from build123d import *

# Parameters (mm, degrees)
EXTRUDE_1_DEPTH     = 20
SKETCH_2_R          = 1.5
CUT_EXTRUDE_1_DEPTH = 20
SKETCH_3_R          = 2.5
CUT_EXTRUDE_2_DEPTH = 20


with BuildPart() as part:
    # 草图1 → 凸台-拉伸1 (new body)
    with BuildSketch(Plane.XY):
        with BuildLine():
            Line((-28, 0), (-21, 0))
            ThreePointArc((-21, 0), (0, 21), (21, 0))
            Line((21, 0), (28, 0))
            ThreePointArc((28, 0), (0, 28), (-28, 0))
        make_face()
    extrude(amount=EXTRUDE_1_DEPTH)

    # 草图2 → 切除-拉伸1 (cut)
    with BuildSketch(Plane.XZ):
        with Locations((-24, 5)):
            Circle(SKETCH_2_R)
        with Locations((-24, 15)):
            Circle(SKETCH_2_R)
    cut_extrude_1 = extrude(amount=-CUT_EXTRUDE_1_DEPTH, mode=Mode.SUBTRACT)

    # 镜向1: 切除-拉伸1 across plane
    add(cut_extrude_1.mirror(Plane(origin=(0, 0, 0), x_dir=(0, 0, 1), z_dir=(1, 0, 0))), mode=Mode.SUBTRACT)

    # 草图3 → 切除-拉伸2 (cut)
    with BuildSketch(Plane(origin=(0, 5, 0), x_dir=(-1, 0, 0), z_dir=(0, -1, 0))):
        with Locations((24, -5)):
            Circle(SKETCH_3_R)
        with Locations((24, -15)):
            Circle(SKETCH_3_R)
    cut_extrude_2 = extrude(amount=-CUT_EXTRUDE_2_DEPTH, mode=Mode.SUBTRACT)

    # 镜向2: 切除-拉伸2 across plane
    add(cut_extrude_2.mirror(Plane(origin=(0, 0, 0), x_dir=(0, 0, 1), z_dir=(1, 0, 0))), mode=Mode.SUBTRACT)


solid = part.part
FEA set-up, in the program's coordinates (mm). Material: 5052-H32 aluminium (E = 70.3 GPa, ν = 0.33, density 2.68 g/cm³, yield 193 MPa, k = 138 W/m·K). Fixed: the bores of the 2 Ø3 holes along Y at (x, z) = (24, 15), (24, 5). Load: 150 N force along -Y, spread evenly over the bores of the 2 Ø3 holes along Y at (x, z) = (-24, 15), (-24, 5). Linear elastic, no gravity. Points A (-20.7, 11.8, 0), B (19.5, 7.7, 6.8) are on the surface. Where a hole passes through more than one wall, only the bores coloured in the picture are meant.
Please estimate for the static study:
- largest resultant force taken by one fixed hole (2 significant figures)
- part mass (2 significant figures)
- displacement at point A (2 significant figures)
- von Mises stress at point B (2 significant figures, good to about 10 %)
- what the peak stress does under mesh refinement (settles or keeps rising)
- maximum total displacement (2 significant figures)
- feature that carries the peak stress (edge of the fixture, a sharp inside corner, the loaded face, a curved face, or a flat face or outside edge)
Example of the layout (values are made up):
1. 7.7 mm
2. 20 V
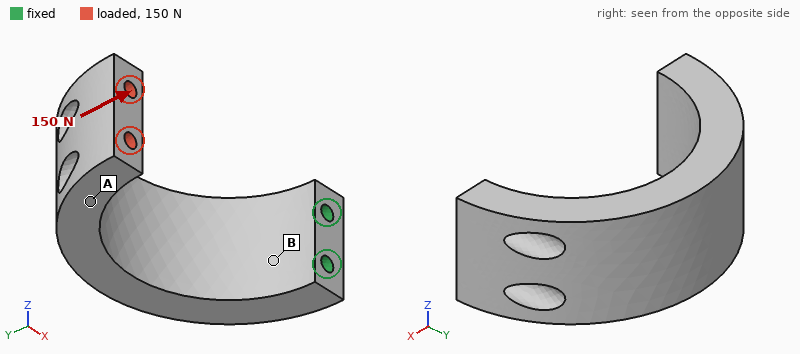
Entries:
1. 110 N
2. 27 g
3. 0.26 mm
4. 56 MPa
5. keeps rising
6. 0.34 mm
7. edge of the fixture
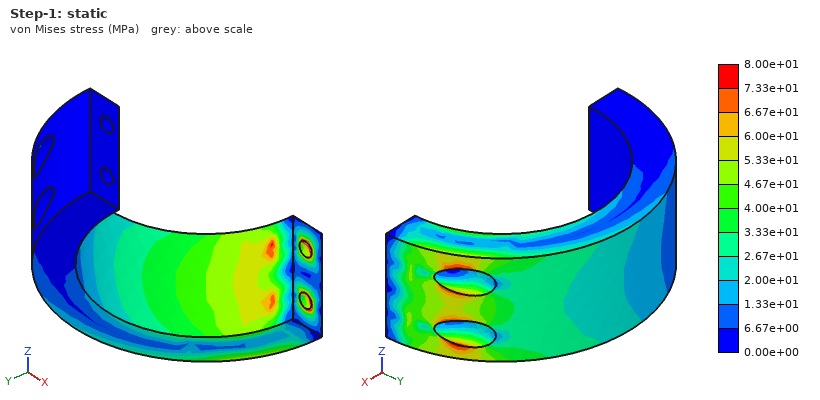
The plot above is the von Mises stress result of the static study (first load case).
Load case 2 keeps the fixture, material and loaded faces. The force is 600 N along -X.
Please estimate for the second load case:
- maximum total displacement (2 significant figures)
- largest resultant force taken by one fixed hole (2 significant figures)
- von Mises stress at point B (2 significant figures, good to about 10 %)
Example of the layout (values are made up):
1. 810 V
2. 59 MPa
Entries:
1. 0.54 mm
2. 310 N
3. 37 MPa
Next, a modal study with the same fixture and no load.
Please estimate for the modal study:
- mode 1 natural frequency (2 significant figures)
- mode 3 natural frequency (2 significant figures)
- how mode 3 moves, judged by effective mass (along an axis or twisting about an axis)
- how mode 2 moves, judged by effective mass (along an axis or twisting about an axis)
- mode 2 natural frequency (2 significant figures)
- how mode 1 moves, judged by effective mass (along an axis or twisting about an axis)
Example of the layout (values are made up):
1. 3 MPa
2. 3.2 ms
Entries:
1. 1200 Hz
2. 3800 Hz
3. along X
4. along Z
5. 1600 Hz
6. along Y
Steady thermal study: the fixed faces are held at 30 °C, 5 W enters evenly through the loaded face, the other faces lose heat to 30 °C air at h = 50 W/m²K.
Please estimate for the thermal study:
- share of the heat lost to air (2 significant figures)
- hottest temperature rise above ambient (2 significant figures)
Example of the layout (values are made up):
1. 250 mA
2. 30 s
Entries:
1. 35 %
2. 16 K
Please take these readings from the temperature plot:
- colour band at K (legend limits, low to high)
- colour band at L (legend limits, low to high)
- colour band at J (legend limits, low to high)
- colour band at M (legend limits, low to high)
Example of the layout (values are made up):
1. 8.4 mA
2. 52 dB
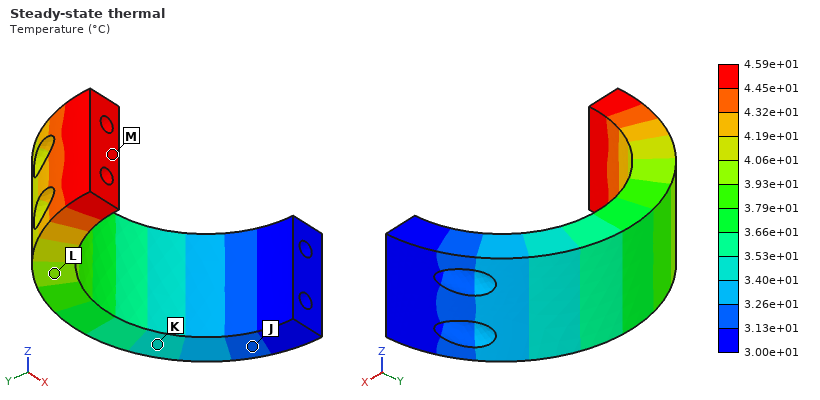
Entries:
1. 3.40e+01 to 3.53e+01 °C
2. 3.93e+01 to 4.06e+01 °C
3. 3.13e+01 to 3.26e+01 °C
4. 4.45e+01 to 4.59e+01 °C
